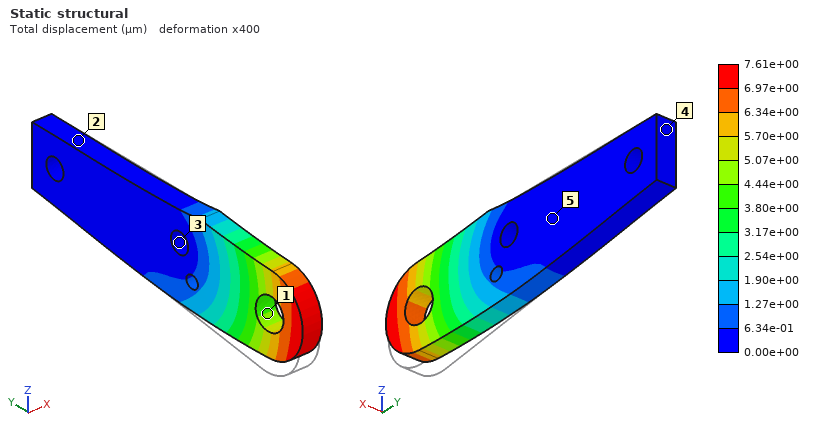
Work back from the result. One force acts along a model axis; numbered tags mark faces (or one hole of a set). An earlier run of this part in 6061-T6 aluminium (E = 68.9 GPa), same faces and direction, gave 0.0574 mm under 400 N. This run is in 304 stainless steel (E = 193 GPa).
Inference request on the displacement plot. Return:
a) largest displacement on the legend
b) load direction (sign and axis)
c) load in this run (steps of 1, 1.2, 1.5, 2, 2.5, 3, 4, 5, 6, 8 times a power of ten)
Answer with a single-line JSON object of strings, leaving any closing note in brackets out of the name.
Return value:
{"largest displacement on the legend": "7.61e+00 µm", "load direction": "+Z", "load in this run": "150 N"}
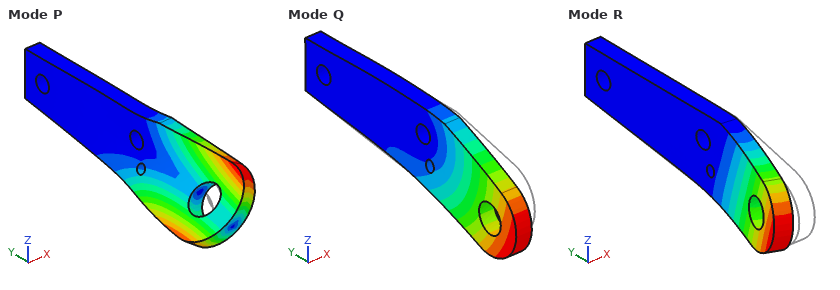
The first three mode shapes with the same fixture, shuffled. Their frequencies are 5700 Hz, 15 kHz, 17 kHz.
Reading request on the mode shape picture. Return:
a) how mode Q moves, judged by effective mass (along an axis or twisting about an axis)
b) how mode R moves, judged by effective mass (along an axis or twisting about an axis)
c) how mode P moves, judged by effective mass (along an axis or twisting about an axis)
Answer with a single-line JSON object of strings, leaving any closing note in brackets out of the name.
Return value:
{"how mode Q moves, judged by effective mass": "along Z", "how mode R moves, judged by effective mass": "along X", "how mode P moves, judged by effective mass": "twisting about Y"}
